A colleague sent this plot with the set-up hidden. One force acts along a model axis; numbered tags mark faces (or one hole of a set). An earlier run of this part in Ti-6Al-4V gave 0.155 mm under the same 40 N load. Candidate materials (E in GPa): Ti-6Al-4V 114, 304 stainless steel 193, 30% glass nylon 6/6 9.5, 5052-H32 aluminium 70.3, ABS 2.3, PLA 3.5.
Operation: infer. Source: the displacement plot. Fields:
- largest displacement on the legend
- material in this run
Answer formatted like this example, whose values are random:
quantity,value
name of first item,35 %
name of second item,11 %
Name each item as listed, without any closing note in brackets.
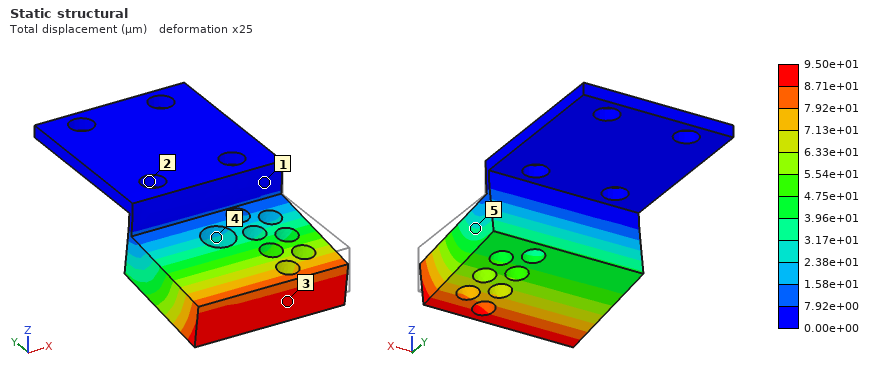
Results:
quantity,value
largest displacement on the legend,9.50e+01 µm
material in this run,304 stainless steel
